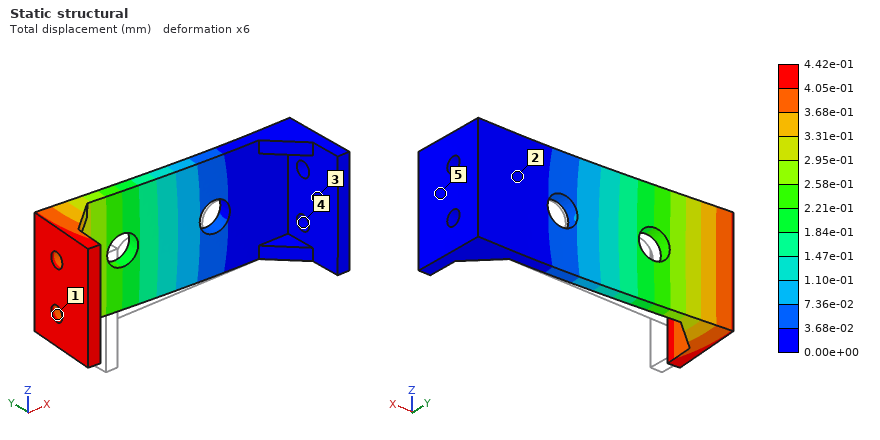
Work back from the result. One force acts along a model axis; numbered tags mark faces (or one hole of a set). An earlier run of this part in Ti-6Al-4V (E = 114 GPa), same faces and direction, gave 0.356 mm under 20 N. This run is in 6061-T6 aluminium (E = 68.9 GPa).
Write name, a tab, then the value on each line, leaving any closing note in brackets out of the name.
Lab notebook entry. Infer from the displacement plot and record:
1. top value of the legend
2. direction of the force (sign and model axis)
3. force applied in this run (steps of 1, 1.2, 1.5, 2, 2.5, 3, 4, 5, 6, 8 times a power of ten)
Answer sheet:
top value of the legend	4.42e-01 mm
direction of the force	+Y
force applied in this run	15 N
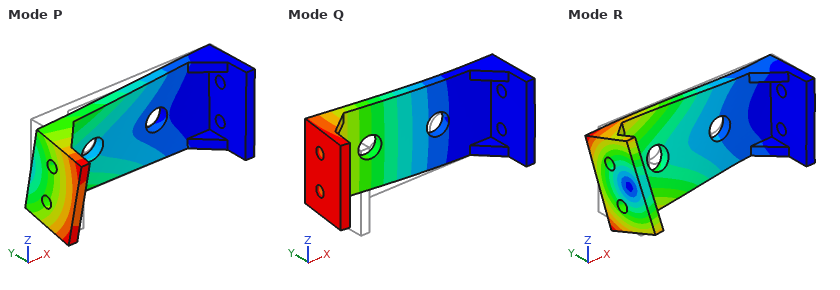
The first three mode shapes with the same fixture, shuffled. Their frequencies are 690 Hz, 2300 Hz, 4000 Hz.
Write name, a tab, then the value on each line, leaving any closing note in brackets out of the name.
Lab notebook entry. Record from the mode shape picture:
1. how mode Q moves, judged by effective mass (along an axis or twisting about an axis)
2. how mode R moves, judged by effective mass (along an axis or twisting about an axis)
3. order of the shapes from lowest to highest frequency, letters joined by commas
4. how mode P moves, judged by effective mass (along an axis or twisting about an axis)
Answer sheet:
how mode Q moves, judged by effective mass	along Y
how mode R moves, judged by effective mass	along Z
order of the shapes from lowest to highest frequency, letters joined by commas	Q, P, R
how mode P moves, judged by effective mass	along Z
